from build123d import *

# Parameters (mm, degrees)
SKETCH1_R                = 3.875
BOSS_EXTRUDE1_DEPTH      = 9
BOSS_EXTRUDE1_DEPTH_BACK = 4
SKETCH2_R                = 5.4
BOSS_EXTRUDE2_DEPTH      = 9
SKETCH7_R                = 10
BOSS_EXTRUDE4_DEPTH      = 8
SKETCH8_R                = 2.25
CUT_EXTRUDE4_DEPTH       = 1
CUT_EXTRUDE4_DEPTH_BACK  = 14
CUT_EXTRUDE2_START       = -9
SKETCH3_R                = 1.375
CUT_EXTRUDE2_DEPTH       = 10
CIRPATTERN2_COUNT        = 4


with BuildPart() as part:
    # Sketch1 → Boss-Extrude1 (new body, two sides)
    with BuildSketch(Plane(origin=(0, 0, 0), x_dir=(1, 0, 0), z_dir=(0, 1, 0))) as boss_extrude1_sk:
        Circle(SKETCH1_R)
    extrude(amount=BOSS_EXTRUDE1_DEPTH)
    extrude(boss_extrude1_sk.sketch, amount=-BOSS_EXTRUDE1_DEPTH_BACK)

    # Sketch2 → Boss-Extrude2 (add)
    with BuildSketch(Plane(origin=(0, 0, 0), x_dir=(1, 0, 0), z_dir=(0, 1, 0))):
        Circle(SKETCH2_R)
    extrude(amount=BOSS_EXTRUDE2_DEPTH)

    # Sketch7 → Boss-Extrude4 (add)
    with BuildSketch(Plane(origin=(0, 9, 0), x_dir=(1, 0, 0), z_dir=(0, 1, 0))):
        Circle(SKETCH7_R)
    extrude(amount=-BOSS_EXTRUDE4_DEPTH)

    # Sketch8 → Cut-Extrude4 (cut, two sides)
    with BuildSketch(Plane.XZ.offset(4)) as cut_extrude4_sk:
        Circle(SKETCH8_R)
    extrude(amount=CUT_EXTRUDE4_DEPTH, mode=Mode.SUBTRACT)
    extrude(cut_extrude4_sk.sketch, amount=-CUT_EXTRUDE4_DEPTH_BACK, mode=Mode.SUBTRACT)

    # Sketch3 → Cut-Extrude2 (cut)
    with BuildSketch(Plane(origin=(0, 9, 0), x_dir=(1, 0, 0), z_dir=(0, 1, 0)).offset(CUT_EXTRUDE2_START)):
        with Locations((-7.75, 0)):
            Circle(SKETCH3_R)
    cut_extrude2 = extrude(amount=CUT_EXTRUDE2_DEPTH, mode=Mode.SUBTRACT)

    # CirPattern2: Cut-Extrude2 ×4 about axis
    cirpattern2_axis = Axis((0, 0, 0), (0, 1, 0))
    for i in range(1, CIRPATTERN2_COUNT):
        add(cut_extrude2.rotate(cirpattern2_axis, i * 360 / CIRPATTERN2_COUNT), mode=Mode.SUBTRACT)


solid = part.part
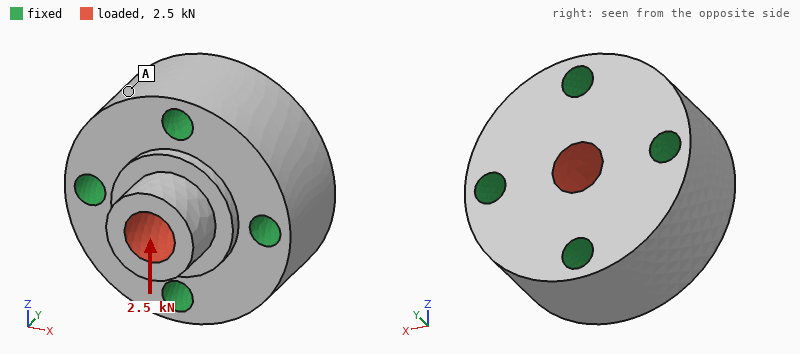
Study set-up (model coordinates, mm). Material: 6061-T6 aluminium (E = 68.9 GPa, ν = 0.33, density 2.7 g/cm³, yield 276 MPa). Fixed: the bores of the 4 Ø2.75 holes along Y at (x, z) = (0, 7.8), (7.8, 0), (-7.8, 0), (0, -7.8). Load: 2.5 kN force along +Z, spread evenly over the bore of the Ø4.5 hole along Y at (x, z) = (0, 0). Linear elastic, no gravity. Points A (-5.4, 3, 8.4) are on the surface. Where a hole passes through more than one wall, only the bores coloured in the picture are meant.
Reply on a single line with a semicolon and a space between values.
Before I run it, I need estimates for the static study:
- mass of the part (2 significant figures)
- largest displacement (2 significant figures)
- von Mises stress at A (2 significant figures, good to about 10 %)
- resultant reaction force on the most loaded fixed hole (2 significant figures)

6.5 g; 8.4 µm; 7.4 MPa; 910 N
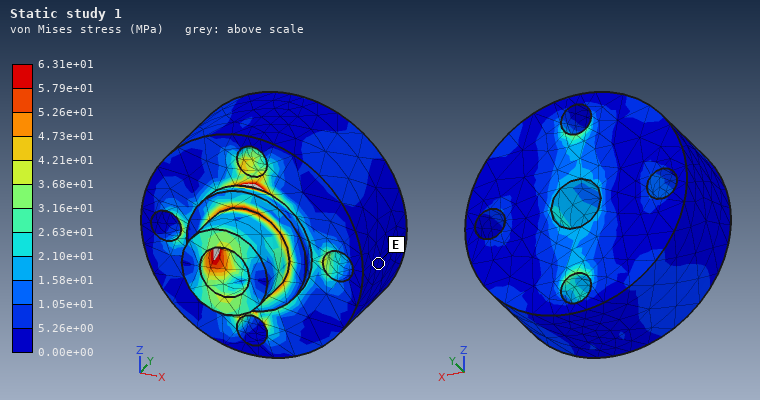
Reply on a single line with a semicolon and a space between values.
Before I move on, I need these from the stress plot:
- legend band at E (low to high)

0.00e+00 to 5.26e+00 MPa
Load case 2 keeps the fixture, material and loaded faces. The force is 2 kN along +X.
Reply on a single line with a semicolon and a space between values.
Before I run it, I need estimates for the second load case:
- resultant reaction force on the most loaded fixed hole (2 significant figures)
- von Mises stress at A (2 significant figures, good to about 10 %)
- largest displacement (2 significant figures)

730 N; 4.6 MPa; 6.7 µm
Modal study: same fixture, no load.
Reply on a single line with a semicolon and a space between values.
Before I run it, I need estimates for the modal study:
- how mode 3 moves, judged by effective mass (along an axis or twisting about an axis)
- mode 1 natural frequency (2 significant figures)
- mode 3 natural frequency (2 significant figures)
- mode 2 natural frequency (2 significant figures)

along Y; 98 kHz; 110 kHz; 98 kHz
